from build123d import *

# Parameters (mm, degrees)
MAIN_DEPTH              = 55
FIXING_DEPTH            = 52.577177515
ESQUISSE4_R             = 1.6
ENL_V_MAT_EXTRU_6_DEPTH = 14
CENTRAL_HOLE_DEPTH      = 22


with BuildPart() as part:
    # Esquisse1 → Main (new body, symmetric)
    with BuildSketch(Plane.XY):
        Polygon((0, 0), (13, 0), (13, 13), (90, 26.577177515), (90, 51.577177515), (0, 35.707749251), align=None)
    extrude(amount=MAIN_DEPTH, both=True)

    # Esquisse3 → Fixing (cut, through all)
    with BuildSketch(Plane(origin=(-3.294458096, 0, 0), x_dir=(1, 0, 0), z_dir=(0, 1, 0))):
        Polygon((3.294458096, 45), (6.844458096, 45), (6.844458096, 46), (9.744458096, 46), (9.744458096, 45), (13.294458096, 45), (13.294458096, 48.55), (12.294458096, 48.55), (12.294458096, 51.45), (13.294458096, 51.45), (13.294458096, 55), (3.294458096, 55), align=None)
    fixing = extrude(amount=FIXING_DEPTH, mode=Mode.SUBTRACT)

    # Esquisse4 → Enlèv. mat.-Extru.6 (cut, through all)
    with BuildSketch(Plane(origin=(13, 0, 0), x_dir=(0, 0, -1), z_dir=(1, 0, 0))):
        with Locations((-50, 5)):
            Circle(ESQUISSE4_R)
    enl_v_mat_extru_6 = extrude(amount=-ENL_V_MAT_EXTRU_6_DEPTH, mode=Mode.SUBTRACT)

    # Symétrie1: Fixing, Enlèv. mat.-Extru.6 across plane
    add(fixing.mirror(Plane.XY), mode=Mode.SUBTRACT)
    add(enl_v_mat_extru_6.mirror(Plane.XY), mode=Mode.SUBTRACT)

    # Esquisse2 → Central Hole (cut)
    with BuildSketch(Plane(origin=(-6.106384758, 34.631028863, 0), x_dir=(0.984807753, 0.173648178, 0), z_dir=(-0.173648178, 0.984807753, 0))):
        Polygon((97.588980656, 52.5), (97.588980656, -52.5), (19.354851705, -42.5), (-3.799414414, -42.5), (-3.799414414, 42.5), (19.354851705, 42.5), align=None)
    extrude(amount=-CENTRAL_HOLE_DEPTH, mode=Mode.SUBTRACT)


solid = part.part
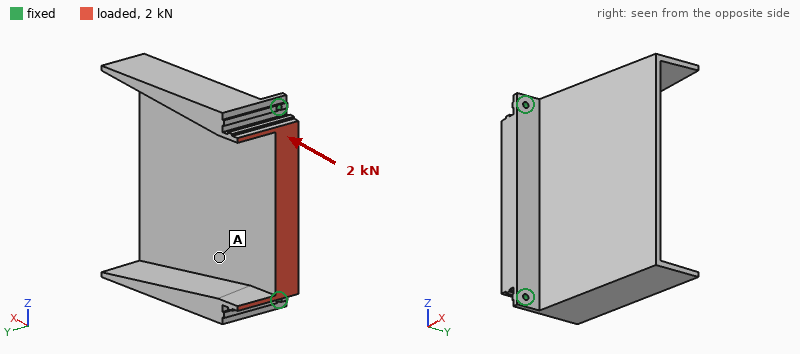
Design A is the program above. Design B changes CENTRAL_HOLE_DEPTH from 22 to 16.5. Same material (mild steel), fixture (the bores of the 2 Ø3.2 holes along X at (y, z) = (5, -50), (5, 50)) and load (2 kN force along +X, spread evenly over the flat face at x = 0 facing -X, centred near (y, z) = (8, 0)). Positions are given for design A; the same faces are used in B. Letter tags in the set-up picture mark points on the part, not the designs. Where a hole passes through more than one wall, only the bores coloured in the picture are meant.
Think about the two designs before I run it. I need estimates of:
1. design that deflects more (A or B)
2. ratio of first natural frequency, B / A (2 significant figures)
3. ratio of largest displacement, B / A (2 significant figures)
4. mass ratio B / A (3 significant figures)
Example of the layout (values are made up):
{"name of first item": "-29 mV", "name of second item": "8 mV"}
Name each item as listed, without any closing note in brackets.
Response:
{"design that deflects more": "B", "ratio of first natural frequency, B / A": "0.76", "ratio of largest displacement, B / A": "2.0", "mass ratio B / A": "1.66"}
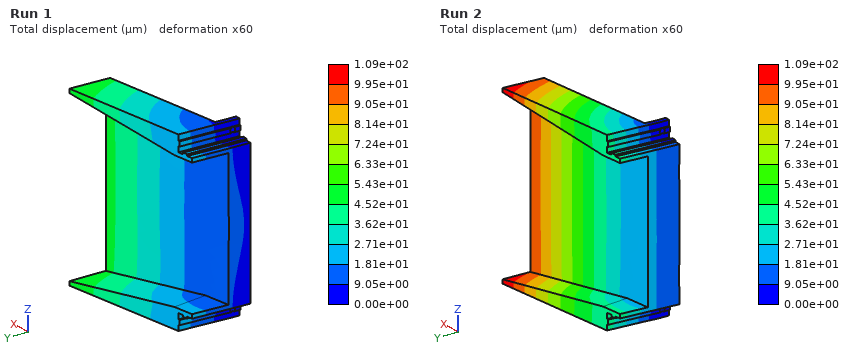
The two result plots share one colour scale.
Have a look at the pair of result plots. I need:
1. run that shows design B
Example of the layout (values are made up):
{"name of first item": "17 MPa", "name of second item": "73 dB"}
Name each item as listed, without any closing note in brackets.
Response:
{"run that shows design B": "Run 2"}
